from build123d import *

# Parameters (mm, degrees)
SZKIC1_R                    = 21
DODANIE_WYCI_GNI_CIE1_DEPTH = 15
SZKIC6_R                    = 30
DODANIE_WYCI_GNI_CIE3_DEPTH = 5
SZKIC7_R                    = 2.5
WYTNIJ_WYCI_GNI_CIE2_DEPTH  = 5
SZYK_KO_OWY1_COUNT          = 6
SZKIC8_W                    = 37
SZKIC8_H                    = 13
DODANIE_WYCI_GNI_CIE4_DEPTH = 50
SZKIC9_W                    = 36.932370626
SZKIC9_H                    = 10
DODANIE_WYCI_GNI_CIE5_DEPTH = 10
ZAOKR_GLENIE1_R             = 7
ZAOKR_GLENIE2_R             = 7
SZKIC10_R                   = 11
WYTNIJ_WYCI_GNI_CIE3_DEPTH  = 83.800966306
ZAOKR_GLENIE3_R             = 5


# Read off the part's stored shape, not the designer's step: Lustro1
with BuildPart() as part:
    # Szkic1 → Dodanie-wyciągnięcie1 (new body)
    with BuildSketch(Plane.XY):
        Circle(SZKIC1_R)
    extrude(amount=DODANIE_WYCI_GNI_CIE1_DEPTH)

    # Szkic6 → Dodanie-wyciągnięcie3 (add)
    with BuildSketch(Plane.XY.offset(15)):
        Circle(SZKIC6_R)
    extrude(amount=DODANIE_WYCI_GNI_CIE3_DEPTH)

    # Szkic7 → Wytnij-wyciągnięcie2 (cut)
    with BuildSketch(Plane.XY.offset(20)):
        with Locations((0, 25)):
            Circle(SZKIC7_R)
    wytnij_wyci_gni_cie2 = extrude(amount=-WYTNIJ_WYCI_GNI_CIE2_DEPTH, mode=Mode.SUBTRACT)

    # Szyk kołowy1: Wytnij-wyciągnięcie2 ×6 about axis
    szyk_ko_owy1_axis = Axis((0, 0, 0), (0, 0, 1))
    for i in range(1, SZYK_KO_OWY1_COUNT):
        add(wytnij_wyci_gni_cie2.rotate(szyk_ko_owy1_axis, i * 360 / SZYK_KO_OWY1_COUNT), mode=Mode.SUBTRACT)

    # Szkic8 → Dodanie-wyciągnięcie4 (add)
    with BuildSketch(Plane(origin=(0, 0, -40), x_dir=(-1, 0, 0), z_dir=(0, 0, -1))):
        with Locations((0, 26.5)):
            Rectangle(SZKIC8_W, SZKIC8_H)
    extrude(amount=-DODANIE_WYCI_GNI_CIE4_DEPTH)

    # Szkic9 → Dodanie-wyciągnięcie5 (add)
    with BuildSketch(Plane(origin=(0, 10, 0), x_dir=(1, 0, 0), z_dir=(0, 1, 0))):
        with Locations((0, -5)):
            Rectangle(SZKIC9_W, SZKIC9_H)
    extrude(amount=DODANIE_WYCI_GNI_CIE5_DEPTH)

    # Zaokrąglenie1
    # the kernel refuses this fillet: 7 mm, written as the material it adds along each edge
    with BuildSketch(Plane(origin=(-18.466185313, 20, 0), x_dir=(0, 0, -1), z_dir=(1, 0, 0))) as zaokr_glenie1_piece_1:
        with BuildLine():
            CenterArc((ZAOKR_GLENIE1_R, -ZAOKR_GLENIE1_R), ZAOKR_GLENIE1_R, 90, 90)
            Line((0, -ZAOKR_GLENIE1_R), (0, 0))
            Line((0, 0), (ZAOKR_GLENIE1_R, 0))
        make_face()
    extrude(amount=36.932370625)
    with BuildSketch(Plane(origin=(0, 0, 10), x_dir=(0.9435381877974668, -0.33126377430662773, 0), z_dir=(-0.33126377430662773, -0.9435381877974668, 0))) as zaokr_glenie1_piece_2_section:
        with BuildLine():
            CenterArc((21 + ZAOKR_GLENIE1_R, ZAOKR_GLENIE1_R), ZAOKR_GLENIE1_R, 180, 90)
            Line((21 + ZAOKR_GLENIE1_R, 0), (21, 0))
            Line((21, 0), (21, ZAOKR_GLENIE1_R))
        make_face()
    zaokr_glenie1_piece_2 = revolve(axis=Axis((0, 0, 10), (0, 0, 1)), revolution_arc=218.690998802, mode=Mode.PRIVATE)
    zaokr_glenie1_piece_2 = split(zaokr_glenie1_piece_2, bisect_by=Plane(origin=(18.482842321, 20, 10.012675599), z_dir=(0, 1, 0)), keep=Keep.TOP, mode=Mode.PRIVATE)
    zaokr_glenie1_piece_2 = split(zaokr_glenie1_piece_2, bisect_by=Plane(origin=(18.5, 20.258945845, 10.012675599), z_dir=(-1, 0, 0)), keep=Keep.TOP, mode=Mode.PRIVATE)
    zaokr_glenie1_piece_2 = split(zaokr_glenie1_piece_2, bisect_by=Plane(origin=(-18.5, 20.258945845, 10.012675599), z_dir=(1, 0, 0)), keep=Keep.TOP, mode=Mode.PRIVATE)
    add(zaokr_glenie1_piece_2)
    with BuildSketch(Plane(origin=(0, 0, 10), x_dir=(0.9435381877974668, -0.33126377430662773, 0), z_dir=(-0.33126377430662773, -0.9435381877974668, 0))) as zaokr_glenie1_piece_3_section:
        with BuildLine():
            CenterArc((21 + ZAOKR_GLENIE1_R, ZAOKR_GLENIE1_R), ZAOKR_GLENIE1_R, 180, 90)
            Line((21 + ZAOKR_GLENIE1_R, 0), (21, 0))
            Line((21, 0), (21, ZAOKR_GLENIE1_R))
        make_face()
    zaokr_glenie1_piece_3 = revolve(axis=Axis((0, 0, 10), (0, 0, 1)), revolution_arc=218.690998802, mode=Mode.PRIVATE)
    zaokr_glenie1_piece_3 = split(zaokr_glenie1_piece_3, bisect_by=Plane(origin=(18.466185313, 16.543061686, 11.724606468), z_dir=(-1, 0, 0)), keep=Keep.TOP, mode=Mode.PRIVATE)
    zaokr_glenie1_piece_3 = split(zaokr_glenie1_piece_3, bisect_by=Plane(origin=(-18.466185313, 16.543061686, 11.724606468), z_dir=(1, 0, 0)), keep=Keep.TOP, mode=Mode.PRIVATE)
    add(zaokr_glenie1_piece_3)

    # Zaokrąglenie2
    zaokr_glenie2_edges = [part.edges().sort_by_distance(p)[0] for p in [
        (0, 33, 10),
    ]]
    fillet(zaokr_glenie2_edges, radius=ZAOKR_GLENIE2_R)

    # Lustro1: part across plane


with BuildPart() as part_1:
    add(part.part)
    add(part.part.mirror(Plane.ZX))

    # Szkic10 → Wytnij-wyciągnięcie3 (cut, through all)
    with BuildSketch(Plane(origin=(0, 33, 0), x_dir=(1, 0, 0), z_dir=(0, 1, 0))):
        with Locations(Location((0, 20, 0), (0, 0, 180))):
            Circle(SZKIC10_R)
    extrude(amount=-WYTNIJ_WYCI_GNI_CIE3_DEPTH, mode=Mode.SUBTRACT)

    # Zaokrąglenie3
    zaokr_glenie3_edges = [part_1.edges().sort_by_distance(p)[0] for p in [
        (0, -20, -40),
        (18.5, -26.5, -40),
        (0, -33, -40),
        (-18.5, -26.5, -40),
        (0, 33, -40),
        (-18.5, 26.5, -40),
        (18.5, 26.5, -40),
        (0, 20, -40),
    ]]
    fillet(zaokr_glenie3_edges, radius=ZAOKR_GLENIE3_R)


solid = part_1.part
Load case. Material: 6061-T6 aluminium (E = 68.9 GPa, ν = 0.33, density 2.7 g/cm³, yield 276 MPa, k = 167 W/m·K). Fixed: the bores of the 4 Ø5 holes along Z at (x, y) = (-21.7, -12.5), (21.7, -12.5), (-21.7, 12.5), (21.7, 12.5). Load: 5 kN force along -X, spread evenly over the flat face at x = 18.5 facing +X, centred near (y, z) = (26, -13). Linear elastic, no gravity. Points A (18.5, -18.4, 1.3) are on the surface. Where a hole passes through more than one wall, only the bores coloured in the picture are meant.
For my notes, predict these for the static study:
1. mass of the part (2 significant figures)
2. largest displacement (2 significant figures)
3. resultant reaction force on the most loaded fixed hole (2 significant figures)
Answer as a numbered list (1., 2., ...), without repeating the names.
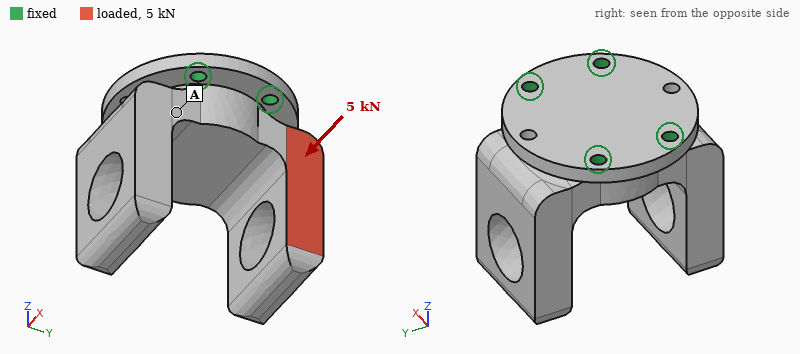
1. 200 g
2. 0.13 mm
3. 3.3 kN
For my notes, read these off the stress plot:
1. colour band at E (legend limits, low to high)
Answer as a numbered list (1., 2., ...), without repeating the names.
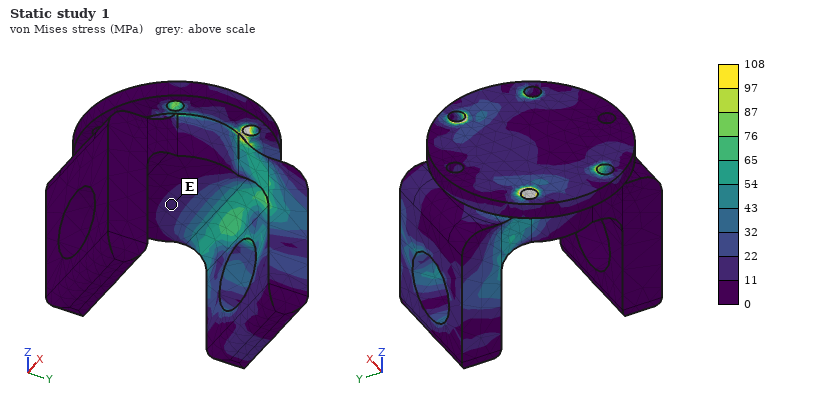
1. 11 to 22 MPa
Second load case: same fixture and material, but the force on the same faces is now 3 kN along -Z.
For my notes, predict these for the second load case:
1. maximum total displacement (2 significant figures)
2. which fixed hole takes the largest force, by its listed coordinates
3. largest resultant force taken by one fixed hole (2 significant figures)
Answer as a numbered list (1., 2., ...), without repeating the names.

1. 0.12 mm
2. (21.7, 12.5)
3. 3.4 kN
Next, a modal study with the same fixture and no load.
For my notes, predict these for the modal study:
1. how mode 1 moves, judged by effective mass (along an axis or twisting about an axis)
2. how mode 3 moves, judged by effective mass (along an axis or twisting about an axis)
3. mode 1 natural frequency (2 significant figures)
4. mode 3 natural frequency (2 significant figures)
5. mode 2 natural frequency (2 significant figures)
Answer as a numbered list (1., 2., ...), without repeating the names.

1. along Y
2. along X
3. 2800 Hz
4. 4700 Hz
5. 3800 Hz
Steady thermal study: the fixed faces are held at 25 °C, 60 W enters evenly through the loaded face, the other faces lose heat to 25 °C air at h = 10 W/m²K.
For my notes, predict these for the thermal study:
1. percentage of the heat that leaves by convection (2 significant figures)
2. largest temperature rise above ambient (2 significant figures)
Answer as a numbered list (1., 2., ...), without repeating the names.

1. 3.6 %
2. 46 K
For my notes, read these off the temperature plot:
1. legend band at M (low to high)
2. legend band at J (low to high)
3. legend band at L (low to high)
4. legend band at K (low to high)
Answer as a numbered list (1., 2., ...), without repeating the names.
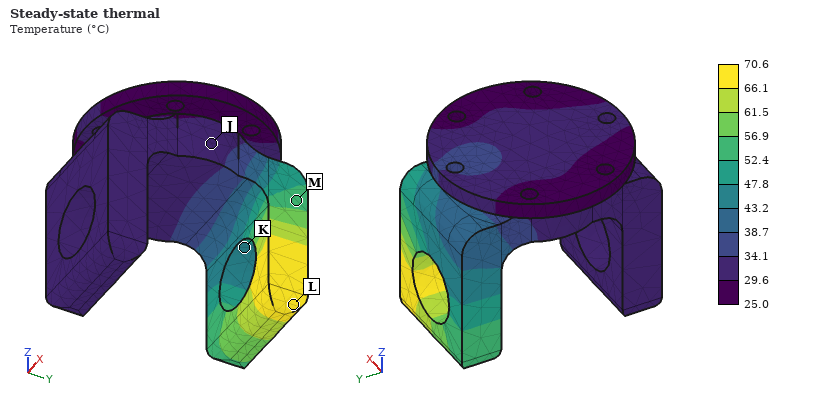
1. 52.4 to 56.9 °C
2. 29.6 to 34.1 °C
3. 66.1 to 70.6 °C
4. 43.2 to 47.8 °C
